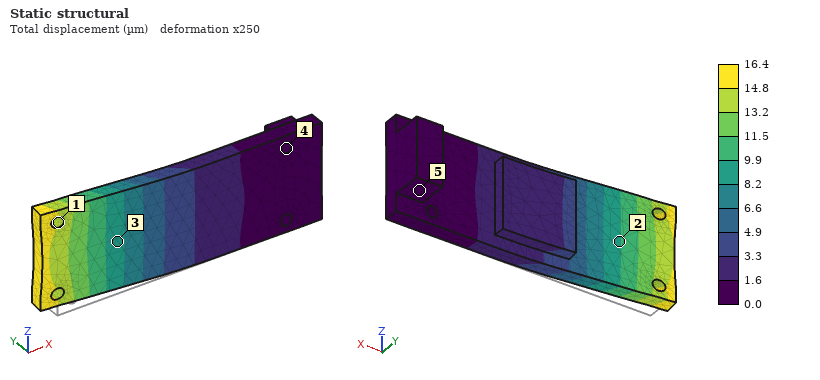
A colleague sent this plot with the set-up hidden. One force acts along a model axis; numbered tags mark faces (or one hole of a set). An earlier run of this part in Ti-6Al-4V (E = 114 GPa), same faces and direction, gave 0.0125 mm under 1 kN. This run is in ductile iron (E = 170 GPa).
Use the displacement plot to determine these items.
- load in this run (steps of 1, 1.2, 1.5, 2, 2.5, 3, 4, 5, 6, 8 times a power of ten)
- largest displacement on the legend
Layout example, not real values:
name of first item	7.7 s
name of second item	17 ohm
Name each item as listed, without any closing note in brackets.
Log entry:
load in this run	2 kN
largest displacement on the legend	16.4 µm
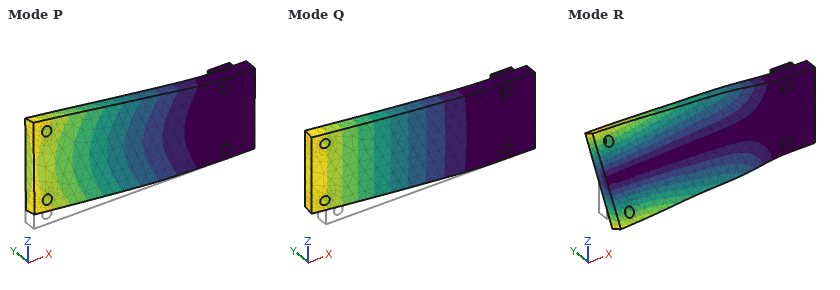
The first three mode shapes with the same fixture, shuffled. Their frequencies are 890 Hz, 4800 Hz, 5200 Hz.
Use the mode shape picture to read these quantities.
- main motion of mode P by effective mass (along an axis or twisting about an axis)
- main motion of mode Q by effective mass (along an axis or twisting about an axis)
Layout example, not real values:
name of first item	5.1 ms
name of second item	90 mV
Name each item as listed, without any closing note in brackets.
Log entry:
main motion of mode P by effective mass	along Z
main motion of mode Q by effective mass	along Y
